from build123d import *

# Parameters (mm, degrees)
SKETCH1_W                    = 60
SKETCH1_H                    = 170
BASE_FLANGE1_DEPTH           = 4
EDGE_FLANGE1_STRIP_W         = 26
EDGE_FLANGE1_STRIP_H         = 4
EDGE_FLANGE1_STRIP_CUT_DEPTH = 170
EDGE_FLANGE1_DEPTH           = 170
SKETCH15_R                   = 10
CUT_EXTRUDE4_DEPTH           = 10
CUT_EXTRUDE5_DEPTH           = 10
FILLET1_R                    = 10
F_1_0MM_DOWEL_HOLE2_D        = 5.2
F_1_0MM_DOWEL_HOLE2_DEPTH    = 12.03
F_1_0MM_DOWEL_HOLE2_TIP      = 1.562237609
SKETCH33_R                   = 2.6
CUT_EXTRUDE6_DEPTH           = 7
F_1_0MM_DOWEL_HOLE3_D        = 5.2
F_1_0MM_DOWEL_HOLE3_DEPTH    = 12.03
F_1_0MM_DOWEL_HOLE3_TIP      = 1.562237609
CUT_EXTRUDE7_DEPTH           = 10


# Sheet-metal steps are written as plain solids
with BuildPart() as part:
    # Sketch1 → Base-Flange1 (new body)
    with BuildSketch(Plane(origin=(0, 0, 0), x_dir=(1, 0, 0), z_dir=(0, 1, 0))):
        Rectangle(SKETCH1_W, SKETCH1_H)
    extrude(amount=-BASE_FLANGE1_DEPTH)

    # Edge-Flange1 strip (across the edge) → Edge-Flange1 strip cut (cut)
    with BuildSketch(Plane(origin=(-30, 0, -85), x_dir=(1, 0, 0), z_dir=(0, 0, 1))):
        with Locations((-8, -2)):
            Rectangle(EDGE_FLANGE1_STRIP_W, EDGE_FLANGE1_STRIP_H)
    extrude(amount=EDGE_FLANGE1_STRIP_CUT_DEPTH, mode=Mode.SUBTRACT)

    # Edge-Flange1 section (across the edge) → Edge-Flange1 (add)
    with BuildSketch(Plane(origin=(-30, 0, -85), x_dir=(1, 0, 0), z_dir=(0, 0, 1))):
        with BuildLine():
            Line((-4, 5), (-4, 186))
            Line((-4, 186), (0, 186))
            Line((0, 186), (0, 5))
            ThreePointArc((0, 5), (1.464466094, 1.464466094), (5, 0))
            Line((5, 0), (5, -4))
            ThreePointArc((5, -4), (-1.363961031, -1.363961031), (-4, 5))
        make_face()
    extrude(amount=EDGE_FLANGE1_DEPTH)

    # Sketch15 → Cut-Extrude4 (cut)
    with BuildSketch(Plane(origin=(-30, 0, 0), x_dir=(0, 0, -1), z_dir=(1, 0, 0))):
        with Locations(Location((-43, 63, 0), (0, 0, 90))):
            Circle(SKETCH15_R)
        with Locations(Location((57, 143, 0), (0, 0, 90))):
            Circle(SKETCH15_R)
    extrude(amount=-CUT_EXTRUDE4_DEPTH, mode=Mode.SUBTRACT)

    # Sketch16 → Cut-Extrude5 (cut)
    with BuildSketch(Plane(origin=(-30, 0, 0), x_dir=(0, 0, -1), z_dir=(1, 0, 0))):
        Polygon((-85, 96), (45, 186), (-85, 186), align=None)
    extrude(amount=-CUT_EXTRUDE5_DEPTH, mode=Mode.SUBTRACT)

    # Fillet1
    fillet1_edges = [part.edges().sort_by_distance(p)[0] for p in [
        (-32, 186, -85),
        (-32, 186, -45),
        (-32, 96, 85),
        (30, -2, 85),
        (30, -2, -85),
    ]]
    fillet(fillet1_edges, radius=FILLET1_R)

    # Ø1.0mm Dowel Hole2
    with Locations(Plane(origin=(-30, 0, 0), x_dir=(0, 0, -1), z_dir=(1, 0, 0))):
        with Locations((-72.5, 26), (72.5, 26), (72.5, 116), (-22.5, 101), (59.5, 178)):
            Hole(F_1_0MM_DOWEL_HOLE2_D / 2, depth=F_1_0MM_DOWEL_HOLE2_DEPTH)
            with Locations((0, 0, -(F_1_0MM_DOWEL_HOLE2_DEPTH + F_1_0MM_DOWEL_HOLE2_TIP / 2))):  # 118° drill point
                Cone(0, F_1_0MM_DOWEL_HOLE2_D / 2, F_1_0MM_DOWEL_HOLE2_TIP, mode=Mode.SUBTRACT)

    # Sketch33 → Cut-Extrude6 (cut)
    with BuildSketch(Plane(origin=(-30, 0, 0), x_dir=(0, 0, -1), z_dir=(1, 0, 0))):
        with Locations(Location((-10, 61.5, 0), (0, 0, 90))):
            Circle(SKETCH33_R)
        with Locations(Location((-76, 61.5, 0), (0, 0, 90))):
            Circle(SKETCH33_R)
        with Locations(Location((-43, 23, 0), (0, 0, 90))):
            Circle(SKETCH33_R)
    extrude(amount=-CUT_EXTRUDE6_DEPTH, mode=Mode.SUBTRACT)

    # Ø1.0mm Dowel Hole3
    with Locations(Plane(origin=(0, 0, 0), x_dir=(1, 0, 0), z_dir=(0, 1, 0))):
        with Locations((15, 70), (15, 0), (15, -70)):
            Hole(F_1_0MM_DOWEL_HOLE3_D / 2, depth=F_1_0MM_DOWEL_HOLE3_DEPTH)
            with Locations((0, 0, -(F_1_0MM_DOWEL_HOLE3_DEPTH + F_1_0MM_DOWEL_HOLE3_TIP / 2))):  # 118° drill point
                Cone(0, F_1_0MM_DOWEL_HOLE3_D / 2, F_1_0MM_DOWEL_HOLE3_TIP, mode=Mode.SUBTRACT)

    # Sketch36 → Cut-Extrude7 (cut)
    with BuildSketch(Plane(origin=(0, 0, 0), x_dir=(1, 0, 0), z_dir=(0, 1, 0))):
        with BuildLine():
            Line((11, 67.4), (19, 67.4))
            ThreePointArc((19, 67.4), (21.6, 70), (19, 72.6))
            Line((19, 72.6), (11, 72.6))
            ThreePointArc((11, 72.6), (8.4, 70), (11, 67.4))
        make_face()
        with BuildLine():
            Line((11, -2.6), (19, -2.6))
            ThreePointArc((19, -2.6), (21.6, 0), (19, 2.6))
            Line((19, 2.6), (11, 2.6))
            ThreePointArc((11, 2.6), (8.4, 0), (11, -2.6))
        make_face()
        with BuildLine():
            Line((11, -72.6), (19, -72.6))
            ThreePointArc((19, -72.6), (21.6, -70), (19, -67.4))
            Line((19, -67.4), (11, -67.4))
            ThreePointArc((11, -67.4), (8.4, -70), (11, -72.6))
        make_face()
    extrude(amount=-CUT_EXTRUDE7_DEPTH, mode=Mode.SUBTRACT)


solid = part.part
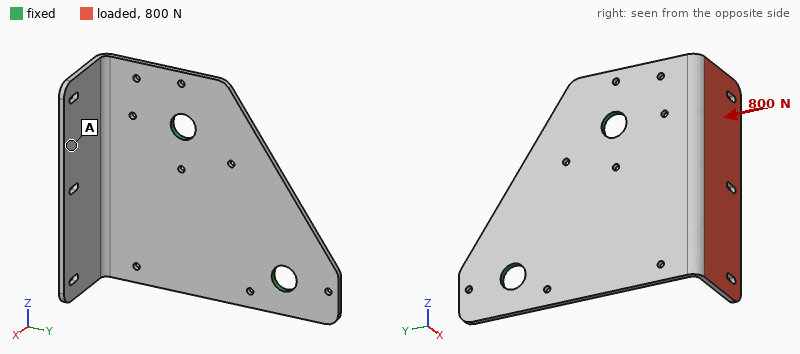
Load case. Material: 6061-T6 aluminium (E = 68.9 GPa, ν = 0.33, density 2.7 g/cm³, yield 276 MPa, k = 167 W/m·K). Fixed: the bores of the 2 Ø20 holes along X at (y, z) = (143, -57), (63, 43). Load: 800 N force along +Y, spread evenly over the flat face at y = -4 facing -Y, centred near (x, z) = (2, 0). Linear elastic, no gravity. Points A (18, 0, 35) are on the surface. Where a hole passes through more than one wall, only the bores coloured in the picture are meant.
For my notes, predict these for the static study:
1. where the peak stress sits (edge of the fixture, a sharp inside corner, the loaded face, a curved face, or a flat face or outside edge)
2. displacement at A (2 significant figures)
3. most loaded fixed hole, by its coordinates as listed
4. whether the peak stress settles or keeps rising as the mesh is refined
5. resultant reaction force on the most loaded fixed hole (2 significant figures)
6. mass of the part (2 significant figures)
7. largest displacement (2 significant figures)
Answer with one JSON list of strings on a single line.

["edge of the fixture", "1.9 mm", "(63, 43)", "keeps rising", "470 N", "380 g", "2.7 mm"]
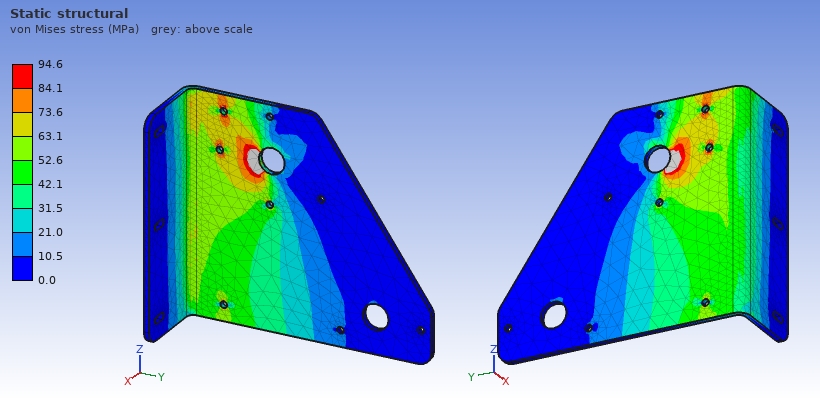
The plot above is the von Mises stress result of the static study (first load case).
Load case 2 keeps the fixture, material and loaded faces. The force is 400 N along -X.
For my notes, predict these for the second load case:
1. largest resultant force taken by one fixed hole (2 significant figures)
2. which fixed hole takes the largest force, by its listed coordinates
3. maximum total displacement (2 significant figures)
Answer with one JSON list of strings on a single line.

["400 N", "(63, 43)", "2.2 mm"]
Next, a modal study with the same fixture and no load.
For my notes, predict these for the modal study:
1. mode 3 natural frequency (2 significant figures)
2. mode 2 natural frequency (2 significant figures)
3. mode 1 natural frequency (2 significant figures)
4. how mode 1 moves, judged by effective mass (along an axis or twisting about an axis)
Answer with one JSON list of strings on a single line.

["660 Hz", "360 Hz", "200 Hz", "along X"]
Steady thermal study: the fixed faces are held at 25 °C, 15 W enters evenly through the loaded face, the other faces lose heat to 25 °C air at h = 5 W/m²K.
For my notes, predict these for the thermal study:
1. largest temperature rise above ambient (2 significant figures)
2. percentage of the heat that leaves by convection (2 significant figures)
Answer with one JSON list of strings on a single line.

["15 K", "12 %"]
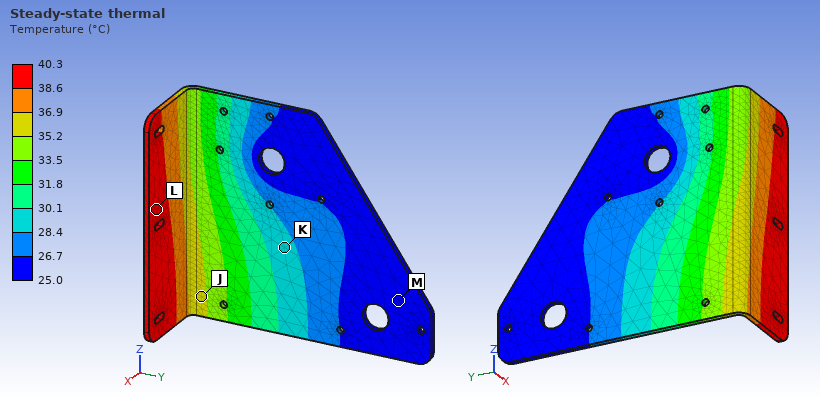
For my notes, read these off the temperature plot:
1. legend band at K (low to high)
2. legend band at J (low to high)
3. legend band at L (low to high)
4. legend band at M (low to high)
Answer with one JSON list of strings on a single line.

["28.4 to 30.1 °C", "35.2 to 36.9 °C", "38.6 to 40.3 °C", "25.0 to 26.7 °C"]
